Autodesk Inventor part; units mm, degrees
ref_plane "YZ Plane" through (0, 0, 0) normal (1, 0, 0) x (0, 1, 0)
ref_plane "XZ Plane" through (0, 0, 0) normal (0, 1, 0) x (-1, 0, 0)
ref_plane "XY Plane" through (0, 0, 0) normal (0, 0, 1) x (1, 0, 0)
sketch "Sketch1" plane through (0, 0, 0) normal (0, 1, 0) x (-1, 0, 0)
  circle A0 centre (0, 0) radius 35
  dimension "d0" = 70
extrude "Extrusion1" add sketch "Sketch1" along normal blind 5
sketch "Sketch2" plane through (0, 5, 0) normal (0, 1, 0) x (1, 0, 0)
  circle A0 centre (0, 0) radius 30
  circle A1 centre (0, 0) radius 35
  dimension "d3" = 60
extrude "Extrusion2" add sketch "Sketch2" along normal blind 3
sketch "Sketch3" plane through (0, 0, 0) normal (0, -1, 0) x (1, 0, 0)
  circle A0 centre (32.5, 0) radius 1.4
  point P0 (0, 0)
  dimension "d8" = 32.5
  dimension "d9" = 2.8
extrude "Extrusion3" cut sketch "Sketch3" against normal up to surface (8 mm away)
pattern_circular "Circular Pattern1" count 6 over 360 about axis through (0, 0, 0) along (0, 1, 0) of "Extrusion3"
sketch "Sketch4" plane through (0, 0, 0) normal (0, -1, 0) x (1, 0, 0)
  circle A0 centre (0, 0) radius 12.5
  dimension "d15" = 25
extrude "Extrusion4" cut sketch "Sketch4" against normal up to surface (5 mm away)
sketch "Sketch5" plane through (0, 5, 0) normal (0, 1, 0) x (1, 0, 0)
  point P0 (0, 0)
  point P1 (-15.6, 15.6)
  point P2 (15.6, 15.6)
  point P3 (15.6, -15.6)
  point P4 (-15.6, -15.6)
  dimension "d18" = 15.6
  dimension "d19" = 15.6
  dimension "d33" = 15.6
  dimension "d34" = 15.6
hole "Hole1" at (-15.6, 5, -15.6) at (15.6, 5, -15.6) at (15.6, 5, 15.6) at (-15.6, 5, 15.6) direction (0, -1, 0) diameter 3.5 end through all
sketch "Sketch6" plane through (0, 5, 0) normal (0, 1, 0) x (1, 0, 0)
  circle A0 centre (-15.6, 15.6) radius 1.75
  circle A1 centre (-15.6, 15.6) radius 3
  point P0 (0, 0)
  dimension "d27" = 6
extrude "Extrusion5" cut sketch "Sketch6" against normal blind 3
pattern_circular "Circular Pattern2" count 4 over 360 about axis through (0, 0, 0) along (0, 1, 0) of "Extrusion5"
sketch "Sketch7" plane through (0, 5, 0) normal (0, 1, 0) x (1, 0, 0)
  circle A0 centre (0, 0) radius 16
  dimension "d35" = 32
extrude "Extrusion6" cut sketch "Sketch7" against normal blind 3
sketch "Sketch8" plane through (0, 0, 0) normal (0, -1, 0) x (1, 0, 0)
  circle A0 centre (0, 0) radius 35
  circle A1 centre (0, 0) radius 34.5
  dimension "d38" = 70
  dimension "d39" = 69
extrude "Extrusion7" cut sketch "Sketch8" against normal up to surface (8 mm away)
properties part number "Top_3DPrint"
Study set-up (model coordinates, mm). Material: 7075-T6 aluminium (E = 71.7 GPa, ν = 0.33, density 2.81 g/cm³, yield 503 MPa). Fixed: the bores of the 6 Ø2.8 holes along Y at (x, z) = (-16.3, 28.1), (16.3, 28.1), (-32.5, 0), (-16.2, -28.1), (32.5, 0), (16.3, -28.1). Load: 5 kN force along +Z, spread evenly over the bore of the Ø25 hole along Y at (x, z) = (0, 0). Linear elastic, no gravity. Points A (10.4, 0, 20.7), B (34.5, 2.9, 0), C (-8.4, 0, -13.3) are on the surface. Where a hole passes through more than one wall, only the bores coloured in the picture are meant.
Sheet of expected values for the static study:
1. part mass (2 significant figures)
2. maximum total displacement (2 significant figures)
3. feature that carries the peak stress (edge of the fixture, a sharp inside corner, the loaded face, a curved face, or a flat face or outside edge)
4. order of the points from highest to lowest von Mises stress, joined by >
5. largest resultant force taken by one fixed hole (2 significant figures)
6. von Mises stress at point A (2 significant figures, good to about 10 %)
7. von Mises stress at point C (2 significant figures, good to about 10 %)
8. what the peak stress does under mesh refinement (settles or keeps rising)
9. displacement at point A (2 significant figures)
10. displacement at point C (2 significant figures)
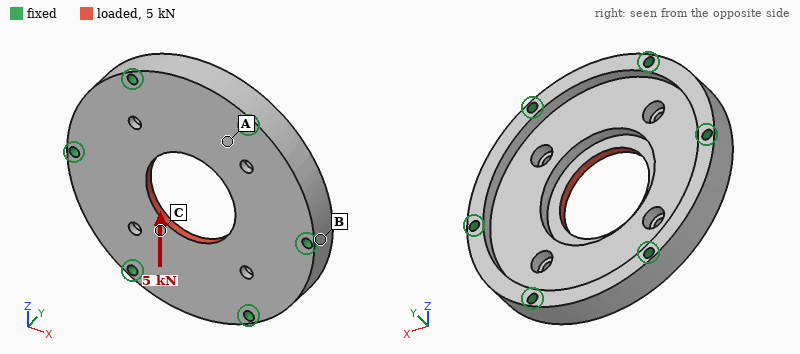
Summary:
49 g
15 µm
edge of the fixture
C > A > B
1.0 kN
27 MPa
35 MPa
keeps rising
4.6 µm
9.5 µm
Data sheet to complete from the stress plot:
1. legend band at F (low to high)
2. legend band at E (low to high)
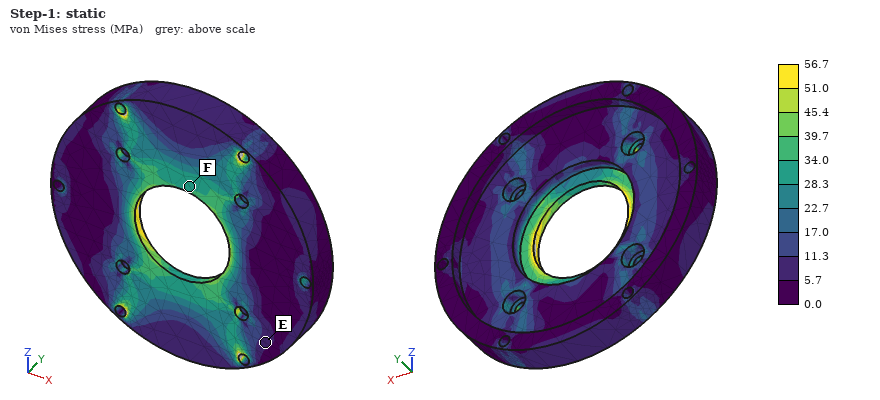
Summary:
28.3 to 34.0 MPa
5.7 to 11.3 MPa
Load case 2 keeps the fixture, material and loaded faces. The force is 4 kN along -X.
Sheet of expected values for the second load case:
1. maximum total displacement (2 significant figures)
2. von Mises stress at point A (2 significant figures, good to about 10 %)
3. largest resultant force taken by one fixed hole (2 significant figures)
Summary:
11 µm
11 MPa
930 N
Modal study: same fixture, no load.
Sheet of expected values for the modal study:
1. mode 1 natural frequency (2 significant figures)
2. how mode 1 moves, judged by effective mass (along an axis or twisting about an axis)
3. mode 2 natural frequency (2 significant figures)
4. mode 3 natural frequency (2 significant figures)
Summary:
13 kHz
along Y
16 kHz
16 kHz
